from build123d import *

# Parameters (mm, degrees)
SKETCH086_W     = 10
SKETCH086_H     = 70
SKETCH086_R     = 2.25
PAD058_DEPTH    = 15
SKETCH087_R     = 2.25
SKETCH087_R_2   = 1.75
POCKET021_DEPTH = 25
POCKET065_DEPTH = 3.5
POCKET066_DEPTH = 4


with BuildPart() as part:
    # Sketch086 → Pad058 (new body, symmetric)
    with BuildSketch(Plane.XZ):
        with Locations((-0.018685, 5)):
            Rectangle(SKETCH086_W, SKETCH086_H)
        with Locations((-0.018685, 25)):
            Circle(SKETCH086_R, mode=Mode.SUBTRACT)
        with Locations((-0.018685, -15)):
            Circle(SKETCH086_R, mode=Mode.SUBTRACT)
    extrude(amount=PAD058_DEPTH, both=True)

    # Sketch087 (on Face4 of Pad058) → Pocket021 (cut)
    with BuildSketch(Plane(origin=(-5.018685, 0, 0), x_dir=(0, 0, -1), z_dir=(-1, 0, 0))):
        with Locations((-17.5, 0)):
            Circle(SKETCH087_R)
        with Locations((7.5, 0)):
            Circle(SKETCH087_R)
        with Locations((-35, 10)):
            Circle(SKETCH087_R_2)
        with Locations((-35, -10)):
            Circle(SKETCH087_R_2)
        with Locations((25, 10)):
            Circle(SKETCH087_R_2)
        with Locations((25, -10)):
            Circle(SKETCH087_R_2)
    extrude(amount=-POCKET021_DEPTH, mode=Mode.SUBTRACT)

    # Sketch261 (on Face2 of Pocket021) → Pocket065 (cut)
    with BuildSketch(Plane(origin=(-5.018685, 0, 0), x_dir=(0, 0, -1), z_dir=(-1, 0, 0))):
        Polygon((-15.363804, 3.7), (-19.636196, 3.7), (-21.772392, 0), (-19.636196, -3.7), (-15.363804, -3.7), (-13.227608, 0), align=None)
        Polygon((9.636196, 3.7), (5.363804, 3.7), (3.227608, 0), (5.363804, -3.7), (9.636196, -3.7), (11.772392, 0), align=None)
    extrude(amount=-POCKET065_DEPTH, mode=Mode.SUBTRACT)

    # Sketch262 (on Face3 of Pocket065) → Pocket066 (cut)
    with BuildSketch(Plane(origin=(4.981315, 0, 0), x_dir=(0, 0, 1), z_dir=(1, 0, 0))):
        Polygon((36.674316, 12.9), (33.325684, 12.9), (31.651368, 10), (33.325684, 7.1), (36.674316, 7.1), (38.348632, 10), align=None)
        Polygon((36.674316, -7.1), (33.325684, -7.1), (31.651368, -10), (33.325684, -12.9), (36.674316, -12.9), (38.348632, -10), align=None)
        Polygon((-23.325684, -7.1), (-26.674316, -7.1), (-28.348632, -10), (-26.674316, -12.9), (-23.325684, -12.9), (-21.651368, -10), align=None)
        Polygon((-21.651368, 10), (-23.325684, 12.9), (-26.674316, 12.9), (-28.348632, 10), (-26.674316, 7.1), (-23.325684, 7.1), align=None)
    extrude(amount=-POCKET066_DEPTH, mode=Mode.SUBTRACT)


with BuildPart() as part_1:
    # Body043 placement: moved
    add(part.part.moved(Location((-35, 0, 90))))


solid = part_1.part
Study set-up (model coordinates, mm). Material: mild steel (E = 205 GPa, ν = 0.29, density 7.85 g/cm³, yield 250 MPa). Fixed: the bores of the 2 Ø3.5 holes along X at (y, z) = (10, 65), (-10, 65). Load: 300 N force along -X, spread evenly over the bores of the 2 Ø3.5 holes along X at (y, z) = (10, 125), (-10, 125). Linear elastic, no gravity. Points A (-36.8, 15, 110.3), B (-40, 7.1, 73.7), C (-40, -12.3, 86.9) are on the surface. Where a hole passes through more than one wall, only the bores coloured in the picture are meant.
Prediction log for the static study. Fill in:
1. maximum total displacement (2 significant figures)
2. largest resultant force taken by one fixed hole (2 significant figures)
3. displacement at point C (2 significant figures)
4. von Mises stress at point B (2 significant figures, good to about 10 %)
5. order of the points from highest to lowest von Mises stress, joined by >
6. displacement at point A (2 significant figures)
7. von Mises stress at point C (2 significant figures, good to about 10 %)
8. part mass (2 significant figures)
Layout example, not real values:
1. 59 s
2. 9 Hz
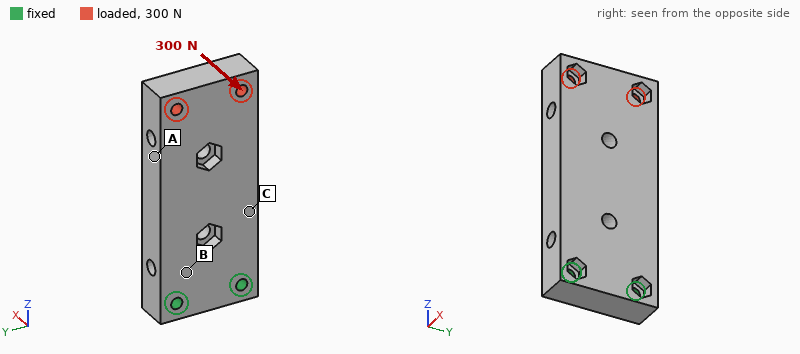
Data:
1. 80 µm
2. 150 N
3. 17 µm
4. 37 MPa
5. B > C > A
6. 48 µm
7. 26 MPa
8. 150 g
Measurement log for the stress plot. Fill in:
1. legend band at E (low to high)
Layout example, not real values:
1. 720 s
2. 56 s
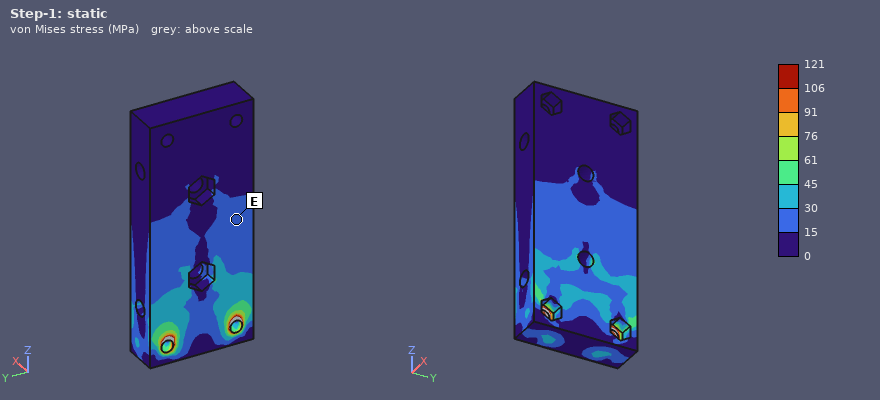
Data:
1. 15 to 30 MPa
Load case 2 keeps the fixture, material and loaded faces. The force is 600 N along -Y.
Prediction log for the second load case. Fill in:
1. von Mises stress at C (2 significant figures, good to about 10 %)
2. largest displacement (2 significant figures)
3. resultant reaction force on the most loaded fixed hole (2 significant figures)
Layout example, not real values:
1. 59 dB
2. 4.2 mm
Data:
1. 14 MPa
2. 20 µm
3. 1.7 kN
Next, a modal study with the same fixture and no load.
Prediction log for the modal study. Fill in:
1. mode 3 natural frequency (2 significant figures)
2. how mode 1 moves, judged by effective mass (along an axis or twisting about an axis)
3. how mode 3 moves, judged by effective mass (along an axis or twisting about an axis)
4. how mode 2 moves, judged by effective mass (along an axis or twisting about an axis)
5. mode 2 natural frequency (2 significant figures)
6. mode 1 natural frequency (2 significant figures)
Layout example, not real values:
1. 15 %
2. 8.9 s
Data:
1. 7000 Hz
2. along X
3. twisting about Z
4. along Y
5. 4400 Hz
6. 1500 Hz
